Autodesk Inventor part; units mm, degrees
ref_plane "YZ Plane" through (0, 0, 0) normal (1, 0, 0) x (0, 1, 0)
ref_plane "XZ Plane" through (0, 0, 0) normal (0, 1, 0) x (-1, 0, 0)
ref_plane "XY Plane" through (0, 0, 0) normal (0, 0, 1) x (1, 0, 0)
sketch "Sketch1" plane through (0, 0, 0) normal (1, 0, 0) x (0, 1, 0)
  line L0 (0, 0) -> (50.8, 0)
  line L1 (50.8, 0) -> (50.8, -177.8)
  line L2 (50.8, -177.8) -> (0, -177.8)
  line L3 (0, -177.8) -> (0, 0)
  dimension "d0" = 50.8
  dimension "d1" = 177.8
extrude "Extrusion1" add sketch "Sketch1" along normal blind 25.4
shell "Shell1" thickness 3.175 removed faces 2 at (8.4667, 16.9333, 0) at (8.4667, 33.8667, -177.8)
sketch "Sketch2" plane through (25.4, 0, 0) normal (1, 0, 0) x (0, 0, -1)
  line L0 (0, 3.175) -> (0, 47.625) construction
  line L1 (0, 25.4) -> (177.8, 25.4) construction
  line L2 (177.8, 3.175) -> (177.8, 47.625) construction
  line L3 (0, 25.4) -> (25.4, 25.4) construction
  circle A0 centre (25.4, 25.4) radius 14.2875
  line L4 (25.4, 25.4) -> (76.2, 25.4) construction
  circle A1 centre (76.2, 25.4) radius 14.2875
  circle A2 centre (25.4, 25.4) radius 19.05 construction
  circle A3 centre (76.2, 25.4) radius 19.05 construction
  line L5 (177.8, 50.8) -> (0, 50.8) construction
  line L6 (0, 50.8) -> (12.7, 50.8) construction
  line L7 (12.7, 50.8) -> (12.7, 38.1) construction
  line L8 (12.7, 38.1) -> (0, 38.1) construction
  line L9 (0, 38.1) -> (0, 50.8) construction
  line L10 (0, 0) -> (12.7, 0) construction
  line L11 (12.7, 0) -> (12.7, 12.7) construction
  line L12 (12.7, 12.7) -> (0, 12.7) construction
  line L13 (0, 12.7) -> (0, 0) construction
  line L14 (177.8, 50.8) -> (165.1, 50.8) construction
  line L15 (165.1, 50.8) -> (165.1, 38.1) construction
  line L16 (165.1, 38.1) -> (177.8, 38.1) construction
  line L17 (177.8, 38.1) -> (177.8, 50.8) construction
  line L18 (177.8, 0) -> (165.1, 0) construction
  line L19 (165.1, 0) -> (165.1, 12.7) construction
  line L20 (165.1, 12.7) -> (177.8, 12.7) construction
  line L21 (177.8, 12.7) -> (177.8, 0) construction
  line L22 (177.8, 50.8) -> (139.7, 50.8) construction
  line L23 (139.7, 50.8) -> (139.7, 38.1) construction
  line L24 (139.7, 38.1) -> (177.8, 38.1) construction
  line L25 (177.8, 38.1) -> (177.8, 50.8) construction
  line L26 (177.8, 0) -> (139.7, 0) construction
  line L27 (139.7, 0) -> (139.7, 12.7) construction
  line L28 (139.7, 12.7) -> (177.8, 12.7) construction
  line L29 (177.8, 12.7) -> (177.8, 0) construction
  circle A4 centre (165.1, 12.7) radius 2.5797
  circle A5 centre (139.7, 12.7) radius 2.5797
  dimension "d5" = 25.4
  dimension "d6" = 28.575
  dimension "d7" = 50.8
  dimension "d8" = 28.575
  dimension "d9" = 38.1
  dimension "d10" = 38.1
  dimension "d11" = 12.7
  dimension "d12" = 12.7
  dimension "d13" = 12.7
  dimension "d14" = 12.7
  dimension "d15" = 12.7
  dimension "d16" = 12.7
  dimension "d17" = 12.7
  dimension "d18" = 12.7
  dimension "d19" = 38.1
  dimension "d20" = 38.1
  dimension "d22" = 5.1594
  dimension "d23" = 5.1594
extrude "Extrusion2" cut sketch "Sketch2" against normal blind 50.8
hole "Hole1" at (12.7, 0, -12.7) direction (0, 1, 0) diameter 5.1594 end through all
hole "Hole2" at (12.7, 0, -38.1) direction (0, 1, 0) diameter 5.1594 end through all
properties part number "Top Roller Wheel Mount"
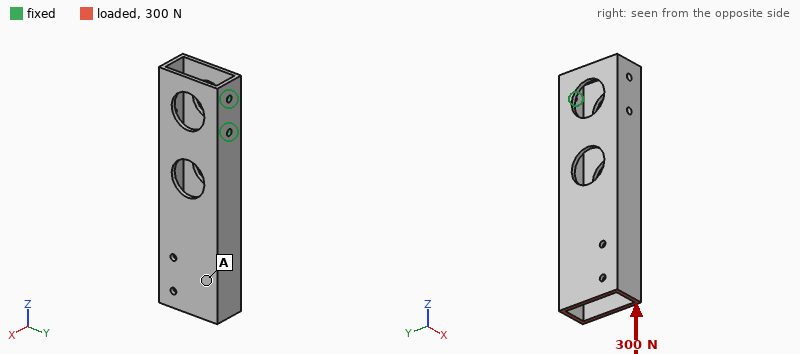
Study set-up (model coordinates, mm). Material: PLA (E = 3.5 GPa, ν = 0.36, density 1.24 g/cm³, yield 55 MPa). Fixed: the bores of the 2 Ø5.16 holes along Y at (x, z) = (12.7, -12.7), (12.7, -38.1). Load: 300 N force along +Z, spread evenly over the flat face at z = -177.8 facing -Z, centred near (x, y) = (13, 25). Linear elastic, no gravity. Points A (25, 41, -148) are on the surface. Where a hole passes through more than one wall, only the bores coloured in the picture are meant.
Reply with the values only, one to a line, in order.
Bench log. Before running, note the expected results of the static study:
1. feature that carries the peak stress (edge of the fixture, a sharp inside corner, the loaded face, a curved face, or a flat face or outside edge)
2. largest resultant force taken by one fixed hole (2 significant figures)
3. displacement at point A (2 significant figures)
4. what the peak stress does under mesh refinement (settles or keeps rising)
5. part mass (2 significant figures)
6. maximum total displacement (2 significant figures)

edge of the fixture
290 N
1.2 mm
keeps rising
87 g
1.6 mm
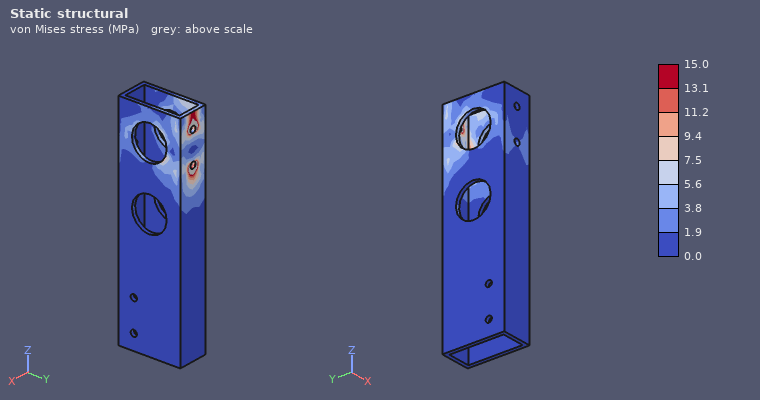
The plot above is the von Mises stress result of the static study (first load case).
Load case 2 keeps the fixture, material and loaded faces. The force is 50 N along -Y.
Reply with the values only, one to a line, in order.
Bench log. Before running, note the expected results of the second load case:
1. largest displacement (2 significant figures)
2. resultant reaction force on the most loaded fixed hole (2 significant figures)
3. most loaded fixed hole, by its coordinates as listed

1.8 mm
270 N
(12.7, -38.1)
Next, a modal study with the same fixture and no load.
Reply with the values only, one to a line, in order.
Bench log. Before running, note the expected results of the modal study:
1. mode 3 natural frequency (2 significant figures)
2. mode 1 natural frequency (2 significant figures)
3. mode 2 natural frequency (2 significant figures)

280 Hz
160 Hz
160 Hz
